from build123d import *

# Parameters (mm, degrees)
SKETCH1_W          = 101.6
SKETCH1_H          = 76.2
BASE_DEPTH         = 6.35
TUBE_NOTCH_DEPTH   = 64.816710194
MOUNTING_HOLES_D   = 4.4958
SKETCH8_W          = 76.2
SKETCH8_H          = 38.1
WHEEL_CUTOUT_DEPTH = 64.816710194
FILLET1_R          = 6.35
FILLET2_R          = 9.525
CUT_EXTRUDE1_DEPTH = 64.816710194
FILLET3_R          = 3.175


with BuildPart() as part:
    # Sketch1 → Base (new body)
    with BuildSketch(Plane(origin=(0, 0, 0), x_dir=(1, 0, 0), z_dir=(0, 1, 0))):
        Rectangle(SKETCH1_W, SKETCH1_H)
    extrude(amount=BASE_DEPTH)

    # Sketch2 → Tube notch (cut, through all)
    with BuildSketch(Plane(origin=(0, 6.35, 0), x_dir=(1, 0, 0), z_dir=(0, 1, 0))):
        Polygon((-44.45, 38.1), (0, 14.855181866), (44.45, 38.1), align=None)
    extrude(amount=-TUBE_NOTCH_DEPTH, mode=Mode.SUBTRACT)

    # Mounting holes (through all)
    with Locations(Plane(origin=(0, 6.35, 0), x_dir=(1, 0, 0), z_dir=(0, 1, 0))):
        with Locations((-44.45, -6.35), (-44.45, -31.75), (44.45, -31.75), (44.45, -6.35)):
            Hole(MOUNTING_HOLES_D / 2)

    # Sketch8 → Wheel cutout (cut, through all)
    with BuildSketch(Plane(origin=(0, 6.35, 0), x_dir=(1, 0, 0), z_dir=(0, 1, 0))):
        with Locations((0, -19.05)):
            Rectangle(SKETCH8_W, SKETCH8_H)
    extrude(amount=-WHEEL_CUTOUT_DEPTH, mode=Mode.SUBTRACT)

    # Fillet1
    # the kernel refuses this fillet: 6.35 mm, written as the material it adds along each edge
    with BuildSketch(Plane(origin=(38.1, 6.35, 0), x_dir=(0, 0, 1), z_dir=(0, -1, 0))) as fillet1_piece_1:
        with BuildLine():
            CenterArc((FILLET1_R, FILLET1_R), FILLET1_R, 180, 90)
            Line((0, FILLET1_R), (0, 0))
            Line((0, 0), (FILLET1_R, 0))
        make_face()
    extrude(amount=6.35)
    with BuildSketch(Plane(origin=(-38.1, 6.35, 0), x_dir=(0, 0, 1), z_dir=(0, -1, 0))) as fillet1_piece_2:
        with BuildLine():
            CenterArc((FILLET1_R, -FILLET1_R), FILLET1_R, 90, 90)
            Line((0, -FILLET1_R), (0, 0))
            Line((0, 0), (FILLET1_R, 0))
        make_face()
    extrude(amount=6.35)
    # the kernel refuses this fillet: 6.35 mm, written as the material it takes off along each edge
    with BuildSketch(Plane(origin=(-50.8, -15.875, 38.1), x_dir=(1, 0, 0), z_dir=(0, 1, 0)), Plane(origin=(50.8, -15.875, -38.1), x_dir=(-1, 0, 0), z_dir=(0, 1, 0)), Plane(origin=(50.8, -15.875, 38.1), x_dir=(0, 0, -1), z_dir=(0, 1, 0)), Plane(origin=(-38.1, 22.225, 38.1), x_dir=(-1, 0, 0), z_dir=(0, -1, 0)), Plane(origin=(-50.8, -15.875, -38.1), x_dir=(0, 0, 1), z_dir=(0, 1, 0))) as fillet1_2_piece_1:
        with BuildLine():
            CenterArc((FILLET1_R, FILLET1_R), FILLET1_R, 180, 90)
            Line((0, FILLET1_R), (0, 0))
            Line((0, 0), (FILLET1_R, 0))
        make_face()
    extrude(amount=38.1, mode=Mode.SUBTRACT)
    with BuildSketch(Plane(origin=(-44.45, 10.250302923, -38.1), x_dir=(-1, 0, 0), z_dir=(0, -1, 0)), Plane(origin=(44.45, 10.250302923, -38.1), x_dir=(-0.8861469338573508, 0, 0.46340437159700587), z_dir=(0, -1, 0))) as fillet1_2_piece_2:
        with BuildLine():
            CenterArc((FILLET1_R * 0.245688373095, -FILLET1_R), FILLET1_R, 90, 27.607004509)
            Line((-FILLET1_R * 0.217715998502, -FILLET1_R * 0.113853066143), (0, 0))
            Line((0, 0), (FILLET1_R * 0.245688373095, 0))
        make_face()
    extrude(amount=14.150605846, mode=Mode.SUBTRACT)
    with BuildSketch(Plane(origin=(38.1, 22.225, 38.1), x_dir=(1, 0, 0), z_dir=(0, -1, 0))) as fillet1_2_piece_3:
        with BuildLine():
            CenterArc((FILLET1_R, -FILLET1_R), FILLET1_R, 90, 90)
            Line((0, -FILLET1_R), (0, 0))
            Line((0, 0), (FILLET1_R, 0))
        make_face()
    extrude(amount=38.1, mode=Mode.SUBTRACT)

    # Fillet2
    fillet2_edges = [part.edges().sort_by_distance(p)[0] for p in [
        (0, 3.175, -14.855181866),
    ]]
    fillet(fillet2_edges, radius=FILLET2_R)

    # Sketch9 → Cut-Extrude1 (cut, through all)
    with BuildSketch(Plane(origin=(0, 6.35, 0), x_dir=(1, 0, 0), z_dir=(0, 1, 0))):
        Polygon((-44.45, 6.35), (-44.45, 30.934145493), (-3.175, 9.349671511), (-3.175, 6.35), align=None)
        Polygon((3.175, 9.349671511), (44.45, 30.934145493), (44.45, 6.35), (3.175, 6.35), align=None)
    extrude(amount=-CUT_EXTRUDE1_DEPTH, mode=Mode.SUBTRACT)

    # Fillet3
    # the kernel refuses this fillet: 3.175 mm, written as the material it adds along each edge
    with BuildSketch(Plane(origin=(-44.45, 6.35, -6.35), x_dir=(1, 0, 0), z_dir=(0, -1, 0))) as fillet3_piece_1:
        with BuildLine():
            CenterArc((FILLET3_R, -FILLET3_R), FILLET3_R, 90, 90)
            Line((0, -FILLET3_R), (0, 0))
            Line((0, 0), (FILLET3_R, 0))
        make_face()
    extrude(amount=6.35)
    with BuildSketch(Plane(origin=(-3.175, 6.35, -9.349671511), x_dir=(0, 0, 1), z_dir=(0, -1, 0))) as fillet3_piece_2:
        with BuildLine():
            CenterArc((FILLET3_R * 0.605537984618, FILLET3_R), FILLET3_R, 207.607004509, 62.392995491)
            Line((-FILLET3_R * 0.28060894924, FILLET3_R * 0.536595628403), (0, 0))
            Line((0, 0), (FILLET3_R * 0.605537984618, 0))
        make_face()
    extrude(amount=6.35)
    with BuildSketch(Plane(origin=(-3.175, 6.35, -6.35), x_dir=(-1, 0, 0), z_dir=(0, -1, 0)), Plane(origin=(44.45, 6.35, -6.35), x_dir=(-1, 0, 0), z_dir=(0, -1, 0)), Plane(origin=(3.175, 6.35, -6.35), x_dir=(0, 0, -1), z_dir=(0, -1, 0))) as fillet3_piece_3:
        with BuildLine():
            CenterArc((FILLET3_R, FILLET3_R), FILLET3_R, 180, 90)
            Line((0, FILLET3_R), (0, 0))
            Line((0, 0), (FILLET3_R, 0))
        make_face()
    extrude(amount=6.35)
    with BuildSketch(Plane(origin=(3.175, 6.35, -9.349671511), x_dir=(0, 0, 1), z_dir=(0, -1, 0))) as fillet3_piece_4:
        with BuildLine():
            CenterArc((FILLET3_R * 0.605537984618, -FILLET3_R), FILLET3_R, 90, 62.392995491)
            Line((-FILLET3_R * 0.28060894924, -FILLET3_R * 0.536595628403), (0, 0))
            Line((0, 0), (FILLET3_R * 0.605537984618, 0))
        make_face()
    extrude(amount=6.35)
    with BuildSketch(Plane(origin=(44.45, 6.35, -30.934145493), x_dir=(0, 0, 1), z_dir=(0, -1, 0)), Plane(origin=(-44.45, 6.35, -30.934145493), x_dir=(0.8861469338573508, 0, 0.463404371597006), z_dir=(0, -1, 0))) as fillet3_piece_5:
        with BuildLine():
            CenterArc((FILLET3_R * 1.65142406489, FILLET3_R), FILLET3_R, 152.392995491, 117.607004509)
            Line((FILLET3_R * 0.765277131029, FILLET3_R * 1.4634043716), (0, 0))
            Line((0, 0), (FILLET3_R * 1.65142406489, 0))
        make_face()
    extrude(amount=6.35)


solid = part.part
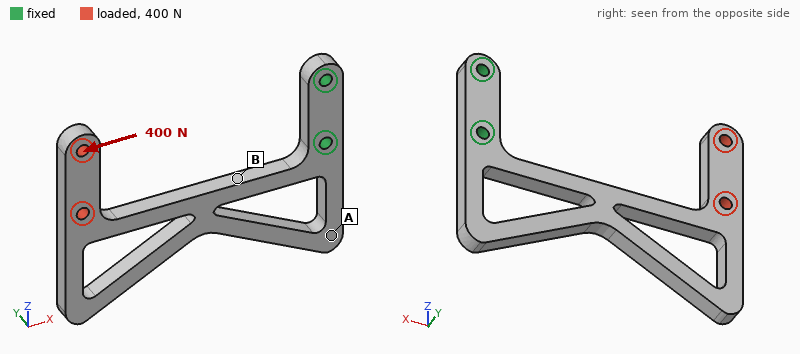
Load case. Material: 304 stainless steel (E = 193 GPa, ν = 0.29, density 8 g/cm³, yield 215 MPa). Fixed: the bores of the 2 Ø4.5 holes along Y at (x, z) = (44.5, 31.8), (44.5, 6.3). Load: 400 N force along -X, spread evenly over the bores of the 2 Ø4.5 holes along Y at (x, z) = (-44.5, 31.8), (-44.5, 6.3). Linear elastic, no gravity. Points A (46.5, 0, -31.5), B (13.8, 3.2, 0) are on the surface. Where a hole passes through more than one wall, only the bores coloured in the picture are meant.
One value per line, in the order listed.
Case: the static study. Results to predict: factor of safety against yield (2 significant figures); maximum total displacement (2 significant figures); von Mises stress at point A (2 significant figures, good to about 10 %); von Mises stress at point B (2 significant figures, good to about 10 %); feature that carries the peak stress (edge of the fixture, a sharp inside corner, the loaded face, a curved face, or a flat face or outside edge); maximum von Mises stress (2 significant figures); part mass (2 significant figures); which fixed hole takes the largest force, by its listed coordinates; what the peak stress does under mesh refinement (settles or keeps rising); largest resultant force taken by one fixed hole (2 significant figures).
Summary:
1.5
0.40 mm
16 MPa
64 MPa
a curved face
150 MPa
130 g
(44.5, 6.3)
settles
310 N
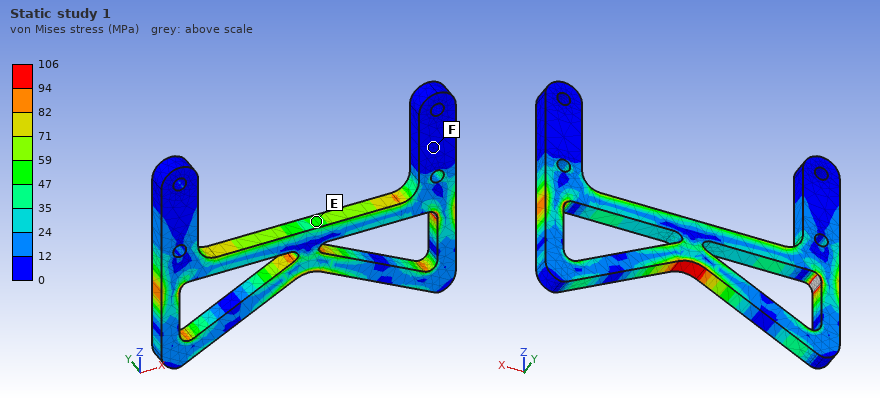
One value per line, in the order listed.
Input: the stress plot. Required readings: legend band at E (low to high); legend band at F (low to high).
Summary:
47 to 59 MPa
0 to 12 MPa
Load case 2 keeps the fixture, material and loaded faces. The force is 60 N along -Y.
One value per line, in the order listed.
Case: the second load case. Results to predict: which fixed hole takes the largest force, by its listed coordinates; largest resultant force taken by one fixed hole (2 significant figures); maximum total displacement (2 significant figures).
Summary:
(44.5, 6.3)
62 N
0.51 mm
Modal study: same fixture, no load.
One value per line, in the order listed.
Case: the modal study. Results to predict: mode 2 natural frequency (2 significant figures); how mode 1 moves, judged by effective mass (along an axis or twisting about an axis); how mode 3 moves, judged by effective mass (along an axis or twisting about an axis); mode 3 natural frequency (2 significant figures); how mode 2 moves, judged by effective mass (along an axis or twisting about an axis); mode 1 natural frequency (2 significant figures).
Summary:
450 Hz
along Y
twisting about X
700 Hz
along Z
290 Hz
